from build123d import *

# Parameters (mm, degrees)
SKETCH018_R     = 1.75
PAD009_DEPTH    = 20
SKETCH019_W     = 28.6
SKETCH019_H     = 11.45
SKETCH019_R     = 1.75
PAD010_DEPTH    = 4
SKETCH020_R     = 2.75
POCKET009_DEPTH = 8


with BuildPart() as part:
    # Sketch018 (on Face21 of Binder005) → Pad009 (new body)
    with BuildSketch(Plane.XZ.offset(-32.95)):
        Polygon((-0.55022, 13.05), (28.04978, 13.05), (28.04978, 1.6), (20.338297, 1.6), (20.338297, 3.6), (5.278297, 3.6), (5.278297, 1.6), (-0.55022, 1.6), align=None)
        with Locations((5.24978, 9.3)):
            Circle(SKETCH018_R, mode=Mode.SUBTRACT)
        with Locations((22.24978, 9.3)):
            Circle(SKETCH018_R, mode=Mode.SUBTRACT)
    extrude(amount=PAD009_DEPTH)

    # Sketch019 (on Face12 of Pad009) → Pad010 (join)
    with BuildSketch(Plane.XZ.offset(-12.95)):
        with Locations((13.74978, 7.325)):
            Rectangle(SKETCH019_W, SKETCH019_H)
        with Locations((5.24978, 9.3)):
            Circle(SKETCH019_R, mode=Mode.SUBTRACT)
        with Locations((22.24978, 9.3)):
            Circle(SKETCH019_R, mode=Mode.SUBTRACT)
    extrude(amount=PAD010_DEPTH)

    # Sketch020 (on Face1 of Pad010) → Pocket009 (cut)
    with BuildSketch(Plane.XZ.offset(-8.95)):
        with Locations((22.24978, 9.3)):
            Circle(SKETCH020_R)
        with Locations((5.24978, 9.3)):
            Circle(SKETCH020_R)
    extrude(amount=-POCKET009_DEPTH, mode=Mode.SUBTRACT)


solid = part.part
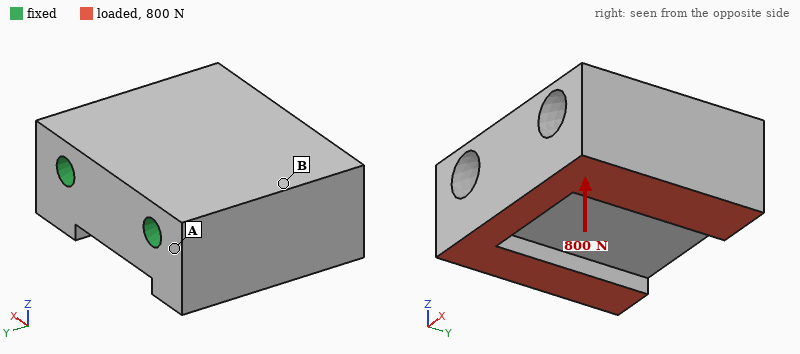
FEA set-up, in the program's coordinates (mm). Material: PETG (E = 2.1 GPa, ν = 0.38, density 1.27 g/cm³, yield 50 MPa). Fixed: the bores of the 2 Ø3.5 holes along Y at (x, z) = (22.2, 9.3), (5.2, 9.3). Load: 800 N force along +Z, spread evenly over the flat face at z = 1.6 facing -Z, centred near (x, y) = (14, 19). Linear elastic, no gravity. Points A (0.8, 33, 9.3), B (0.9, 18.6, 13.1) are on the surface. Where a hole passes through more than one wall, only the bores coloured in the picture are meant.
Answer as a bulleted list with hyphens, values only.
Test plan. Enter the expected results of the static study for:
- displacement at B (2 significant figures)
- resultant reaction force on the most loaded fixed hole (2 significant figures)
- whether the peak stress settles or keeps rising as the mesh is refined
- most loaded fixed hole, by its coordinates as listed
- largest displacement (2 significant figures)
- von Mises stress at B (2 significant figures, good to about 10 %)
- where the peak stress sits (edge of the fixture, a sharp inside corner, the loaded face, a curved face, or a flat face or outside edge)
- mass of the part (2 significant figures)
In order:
- 19 µm
- 430 N
- keeps rising
- (22.2, 9.3)
- 78 µm
- 4.8 MPa
- edge of the fixture
- 8.3 g
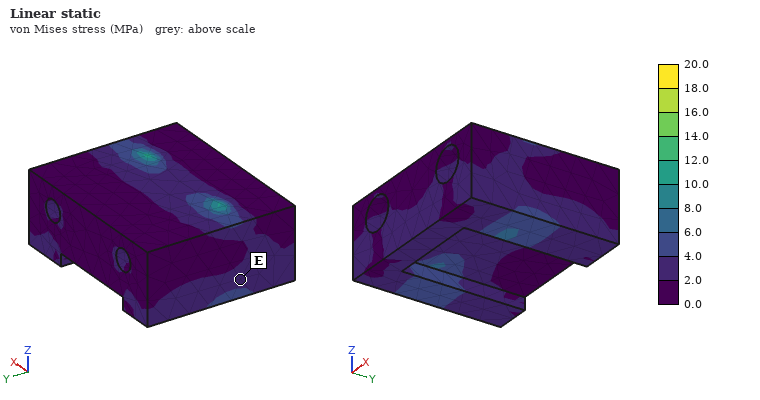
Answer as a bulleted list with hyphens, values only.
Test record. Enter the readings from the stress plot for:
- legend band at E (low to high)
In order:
- 2.0 to 4.0 MPa
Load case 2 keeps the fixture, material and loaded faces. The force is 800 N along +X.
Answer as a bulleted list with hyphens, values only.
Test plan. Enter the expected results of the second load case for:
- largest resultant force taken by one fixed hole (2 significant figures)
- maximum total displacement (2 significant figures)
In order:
- 490 N
- 86 µm
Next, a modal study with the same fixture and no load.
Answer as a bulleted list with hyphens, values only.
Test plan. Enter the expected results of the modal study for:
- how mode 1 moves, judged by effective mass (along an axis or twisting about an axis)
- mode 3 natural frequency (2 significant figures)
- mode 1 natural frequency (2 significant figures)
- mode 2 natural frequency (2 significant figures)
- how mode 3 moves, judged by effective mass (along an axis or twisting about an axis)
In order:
- along Z
- 12 kHz
- 8200 Hz
- 11 kHz
- along X
